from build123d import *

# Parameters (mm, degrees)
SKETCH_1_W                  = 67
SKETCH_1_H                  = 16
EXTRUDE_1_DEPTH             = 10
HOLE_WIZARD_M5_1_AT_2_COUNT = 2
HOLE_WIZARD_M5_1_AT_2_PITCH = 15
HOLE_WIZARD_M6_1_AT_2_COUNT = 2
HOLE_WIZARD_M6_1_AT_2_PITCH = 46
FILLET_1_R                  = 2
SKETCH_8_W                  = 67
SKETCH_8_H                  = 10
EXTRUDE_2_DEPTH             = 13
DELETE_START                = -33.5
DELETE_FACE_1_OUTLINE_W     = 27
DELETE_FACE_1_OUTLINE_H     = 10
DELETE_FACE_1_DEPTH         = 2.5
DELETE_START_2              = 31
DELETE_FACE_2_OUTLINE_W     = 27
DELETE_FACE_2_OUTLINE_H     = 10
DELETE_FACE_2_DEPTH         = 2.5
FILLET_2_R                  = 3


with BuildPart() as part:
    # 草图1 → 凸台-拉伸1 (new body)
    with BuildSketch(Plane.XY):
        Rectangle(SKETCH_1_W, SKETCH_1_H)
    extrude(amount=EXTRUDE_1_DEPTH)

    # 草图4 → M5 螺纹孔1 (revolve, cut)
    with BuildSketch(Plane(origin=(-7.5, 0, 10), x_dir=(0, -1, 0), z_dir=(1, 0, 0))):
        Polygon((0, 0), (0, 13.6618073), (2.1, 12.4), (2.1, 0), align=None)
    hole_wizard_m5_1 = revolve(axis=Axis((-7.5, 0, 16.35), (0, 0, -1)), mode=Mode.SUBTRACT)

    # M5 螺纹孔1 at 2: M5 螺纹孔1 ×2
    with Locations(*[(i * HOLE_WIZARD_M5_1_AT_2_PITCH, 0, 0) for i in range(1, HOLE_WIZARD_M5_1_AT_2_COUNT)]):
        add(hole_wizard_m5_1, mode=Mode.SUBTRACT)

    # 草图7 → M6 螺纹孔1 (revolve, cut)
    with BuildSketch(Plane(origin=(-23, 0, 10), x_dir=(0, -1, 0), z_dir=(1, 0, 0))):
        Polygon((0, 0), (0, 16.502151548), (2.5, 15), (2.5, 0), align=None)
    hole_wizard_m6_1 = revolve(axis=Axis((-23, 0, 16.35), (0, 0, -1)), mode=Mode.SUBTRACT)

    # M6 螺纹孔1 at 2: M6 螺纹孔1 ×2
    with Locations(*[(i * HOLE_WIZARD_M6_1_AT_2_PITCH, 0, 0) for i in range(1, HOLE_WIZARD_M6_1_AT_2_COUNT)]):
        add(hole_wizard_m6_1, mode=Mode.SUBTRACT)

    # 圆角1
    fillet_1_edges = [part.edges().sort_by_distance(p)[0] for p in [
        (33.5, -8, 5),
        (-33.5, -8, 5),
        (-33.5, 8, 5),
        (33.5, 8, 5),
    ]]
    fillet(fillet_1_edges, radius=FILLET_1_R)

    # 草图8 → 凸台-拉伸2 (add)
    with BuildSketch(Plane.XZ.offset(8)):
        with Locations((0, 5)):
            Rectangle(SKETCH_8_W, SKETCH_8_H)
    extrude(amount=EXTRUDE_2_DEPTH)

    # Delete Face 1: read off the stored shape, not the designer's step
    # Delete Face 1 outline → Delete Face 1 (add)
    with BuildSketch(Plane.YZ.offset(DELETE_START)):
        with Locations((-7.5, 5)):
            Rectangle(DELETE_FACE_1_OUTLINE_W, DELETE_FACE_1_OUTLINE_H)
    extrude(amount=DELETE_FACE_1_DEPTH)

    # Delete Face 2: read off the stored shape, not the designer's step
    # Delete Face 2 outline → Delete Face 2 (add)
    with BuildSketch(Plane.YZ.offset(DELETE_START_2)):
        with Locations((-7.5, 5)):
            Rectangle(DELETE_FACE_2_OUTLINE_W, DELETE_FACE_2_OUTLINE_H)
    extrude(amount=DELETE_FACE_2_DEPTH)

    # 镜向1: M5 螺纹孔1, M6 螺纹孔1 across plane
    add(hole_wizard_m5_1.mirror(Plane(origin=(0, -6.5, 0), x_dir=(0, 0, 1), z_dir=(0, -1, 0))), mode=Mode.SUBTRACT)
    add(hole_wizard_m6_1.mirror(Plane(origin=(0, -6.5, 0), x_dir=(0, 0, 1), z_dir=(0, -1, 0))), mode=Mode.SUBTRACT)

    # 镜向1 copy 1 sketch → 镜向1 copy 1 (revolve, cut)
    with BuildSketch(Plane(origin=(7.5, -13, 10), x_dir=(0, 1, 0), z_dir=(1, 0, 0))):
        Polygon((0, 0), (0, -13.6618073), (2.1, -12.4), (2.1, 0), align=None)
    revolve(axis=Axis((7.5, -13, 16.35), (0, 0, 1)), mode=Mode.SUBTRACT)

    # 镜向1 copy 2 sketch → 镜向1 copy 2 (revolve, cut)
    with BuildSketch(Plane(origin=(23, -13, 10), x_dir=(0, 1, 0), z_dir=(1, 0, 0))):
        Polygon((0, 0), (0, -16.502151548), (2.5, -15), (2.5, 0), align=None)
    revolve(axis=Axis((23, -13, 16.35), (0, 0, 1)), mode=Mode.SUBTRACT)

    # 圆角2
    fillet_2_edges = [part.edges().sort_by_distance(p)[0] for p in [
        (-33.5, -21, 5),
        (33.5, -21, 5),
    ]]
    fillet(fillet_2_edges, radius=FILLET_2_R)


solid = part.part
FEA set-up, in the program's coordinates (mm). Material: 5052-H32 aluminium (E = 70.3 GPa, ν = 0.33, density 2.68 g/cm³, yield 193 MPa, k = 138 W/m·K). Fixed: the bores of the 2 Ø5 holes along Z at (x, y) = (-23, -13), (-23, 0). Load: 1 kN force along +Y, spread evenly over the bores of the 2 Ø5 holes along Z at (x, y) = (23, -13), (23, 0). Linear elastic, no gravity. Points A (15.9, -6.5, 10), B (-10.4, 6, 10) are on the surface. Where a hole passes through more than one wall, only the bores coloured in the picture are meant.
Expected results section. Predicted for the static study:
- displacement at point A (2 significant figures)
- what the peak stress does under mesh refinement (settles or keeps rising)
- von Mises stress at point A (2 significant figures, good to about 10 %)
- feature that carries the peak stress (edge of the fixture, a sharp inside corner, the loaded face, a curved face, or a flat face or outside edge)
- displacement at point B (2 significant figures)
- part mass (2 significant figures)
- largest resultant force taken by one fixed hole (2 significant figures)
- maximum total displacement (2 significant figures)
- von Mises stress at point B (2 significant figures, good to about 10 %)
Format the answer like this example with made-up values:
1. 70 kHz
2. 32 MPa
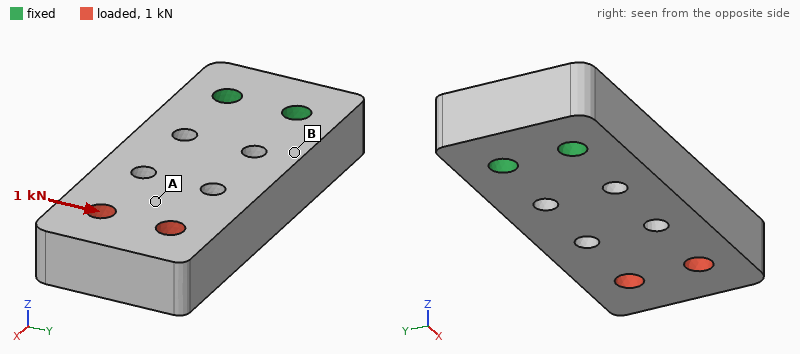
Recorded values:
1. 30 µm
2. keeps rising
3. 6.5 MPa
4. edge of the fixture
5. 8.6 µm
6. 48 g
7. 2.8 kN
8. 48 µm
9. 24 MPa
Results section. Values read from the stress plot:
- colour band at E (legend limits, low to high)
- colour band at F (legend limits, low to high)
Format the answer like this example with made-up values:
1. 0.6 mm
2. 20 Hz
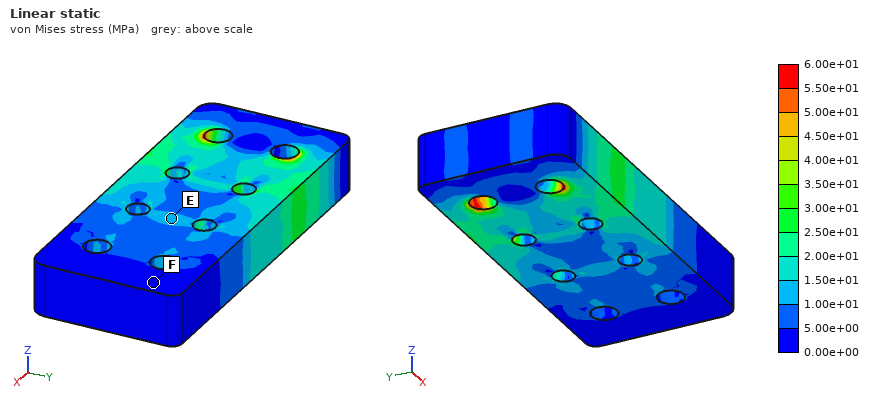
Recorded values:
1. 1.00e+01 to 1.50e+01 MPa
2. 0.00e+00 to 5.00e+00 MPa
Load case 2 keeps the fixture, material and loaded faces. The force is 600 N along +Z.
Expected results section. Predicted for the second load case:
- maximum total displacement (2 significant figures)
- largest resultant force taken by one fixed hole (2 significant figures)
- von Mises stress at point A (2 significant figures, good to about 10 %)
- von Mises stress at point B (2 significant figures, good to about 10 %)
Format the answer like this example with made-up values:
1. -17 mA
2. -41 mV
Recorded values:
1. 0.17 mm
2. 300 N
3. 11 MPa
4. 49 MPa
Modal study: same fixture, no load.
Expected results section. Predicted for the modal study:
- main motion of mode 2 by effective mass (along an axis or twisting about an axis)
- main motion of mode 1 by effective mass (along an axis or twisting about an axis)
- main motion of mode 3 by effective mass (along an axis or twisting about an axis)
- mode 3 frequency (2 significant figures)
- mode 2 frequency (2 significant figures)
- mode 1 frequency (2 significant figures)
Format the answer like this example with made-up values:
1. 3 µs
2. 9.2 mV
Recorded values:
1. along Y
2. along Z
3. twisting about X
4. 8500 Hz
5. 5900 Hz
6. 2600 Hz
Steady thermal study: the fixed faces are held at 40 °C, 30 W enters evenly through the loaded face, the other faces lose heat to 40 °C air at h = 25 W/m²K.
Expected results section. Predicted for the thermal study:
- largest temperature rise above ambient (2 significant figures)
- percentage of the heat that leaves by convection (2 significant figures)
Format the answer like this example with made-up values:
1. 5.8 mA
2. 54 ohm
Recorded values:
1. 37 K
2. 8.6 %
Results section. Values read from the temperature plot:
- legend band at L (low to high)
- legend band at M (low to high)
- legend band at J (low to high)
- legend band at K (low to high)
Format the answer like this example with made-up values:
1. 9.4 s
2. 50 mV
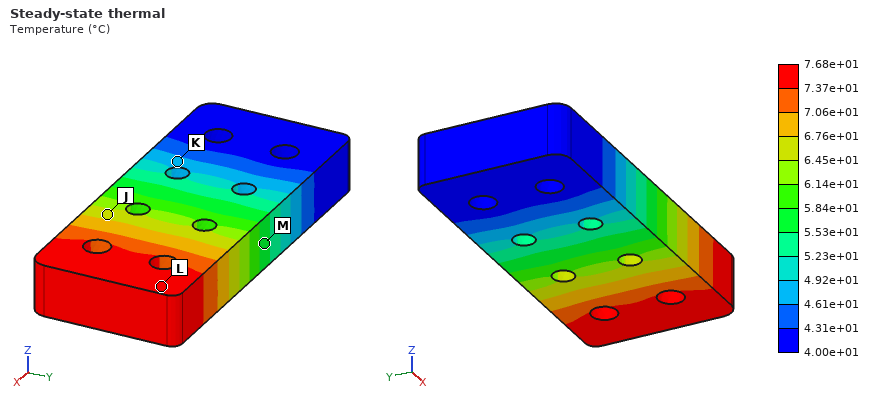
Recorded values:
1. 7.37e+01 to 7.68e+01 °C
2. 5.53e+01 to 5.84e+01 °C
3. 6.45e+01 to 6.76e+01 °C
4. 4.61e+01 to 4.92e+01 °C
